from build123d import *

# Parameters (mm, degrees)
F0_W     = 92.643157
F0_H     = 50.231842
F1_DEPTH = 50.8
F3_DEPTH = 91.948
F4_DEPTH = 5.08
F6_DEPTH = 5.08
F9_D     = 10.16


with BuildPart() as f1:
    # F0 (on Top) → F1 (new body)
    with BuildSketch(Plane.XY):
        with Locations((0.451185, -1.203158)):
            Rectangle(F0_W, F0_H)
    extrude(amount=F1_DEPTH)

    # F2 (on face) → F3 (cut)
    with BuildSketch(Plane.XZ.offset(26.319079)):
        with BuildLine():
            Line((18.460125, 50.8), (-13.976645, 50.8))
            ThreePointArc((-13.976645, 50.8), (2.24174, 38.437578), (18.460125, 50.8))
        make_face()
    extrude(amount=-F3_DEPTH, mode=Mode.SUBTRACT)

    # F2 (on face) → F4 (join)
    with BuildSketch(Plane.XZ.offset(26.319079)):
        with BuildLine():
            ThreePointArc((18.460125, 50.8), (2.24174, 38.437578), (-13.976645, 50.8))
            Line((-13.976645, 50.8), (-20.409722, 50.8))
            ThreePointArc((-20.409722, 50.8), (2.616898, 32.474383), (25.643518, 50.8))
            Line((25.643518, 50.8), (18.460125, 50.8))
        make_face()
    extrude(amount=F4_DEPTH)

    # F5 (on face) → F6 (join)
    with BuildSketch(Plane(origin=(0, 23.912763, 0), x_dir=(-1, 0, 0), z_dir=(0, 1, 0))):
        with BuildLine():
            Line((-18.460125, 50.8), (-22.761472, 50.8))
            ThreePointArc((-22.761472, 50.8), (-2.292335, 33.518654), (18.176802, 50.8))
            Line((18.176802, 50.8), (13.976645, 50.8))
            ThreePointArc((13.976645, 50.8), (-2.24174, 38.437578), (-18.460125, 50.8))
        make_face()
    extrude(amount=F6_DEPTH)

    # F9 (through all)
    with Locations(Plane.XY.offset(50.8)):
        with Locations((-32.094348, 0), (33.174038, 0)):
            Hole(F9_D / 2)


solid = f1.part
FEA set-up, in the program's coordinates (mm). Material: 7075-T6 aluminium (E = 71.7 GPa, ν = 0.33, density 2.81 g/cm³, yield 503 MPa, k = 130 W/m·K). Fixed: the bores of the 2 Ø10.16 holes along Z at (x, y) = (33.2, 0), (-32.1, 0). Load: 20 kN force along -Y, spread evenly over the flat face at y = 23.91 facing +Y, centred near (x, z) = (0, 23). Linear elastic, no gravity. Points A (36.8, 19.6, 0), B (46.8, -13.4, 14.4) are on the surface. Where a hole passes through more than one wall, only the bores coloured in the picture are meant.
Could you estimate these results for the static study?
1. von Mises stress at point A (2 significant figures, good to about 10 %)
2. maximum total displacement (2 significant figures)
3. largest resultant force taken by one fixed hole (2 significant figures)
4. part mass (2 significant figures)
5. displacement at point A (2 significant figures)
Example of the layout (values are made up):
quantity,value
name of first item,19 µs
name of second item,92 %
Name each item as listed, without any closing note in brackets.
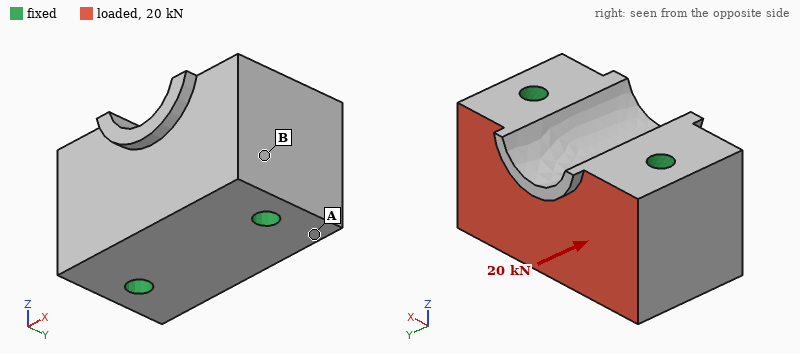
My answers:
quantity,value
von Mises stress at point A,5.2 MPa
maximum total displacement,4.3 µm
largest resultant force taken by one fixed hole,10 kN
part mass,610 g
displacement at point A,1.7 µm
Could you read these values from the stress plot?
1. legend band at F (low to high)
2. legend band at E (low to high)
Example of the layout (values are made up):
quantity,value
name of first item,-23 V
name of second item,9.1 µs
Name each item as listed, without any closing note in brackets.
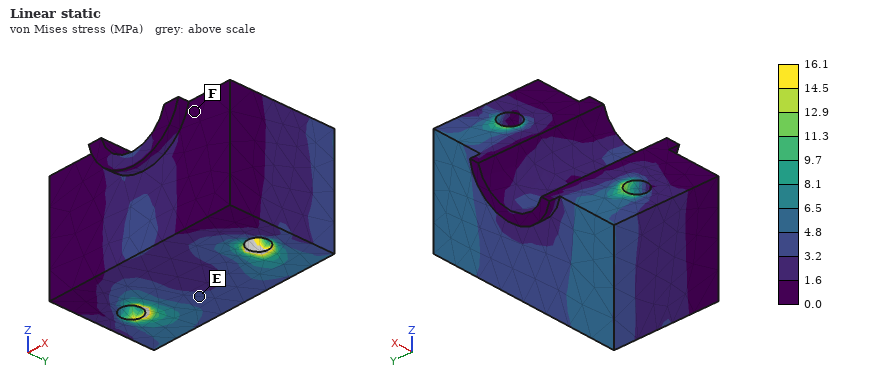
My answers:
quantity,value
legend band at F,0.0 to 1.6 MPa
legend band at E,3.2 to 4.8 MPa
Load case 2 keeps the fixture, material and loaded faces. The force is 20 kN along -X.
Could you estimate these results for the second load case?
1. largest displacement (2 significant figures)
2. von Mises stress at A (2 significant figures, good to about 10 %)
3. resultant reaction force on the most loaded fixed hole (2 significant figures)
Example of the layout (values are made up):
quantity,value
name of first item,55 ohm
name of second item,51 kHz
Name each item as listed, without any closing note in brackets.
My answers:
quantity,value
largest displacement,9.0 µm
von Mises stress at A,8.0 MPa
resultant reaction force on the most loaded fixed hole,12 kN
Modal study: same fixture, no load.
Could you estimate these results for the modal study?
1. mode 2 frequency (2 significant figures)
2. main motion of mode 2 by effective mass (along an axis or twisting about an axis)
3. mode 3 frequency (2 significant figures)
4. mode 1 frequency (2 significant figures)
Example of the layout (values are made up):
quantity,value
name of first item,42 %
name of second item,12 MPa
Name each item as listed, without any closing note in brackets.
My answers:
quantity,value
mode 2 frequency,18 kHz
main motion of mode 2 by effective mass,along Z
mode 3 frequency,20 kHz
mode 1 frequency,18 kHz
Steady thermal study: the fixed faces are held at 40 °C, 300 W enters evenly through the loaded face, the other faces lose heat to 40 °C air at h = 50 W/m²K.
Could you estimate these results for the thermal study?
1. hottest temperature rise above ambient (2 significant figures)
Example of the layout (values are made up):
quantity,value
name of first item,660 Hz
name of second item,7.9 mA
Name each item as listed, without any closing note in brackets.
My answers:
quantity,value
hottest temperature rise above ambient,16 K
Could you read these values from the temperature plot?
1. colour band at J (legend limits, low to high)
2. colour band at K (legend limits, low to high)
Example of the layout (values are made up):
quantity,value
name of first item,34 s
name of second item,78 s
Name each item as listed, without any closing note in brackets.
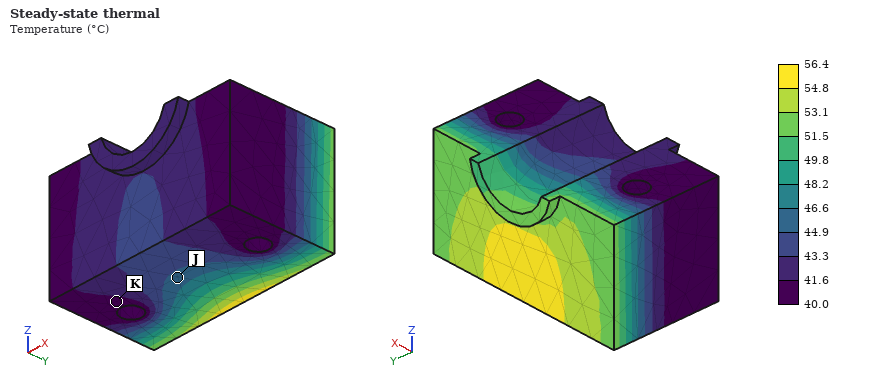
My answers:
quantity,value
colour band at J,44.9 to 46.6 °C
colour band at K,40.0 to 41.6 °C
